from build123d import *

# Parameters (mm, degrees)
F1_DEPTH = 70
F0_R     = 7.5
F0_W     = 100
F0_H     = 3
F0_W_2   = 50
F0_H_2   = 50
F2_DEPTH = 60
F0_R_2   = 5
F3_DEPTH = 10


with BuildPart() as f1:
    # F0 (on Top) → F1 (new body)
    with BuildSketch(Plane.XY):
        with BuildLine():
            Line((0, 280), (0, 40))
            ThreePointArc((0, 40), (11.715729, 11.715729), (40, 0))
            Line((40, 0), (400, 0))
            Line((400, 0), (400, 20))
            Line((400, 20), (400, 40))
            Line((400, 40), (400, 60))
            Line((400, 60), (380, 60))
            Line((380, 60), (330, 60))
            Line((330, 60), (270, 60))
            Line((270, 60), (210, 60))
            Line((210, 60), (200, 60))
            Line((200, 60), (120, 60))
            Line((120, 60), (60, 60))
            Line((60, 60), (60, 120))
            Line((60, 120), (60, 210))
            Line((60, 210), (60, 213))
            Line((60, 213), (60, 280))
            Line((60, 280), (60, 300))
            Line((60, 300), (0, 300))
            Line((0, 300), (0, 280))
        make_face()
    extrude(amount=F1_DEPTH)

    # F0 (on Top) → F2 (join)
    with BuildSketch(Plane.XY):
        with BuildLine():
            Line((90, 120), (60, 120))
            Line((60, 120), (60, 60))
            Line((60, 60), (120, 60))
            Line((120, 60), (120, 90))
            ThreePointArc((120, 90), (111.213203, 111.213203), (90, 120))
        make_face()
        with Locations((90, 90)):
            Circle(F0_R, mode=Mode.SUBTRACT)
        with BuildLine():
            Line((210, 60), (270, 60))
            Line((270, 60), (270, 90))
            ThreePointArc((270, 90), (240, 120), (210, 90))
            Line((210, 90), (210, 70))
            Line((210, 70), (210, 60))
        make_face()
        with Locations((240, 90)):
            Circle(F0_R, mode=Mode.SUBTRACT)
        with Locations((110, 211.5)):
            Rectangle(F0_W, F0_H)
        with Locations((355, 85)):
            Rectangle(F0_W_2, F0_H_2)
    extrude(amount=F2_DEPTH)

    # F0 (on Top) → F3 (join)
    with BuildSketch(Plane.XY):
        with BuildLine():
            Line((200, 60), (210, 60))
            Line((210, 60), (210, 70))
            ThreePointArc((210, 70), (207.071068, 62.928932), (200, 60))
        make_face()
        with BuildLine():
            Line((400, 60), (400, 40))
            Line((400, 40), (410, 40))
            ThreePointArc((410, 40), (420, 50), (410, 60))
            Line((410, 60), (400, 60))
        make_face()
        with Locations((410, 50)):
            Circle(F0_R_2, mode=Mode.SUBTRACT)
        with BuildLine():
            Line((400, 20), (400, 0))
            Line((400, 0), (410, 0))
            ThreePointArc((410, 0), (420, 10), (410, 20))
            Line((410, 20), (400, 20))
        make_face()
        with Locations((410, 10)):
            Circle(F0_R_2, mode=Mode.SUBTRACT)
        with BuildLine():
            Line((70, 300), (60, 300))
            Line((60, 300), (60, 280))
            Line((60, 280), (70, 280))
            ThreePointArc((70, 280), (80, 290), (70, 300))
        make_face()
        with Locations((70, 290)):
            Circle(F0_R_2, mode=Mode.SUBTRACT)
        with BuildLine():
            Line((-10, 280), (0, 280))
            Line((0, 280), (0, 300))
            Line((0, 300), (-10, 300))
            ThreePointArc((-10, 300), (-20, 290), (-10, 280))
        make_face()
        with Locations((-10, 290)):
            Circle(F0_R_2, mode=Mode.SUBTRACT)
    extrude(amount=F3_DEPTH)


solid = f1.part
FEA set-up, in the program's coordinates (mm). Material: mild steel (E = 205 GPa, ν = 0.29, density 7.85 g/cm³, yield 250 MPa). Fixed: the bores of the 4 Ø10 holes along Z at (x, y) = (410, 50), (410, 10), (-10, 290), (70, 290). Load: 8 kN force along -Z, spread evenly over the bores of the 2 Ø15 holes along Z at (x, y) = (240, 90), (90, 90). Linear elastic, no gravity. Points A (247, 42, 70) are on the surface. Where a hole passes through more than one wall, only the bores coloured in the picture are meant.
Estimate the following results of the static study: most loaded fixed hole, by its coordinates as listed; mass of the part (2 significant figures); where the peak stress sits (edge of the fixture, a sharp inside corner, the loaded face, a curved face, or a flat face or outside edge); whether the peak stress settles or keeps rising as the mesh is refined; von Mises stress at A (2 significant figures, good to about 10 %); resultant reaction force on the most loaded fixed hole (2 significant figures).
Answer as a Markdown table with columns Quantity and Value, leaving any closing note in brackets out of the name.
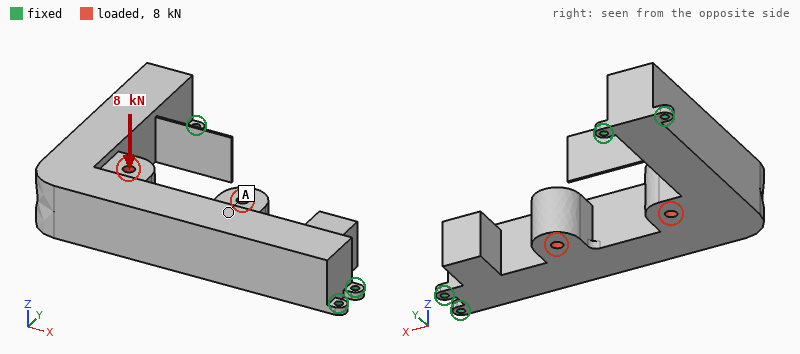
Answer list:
| Quantity | Value |
|---|---|
| most loaded fixed hole, by its coordinates as listed | (410, 10) |
| mass of the part | 25 kg |
| where the peak stress sits | edge of the fixture |
| whether the peak stress settles or keeps rising as the mesh is refined | keeps rising |
| von Mises stress at A | 14 MPa |
| resultant reaction force on the most loaded fixed hole | 13 kN |
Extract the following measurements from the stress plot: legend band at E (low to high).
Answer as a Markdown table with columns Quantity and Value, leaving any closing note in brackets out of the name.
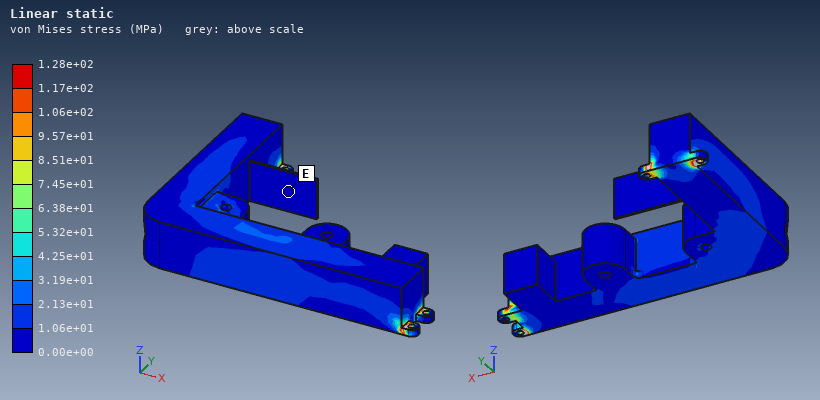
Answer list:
| Quantity | Value |
|---|---|
| legend band at E | 0.00e+00 to 1.06e+01 MPa |
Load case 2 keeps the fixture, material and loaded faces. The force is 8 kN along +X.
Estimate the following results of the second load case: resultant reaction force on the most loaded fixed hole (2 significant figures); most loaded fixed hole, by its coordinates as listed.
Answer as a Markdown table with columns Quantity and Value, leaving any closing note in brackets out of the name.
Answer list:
| Quantity | Value |
|---|---|
| resultant reaction force on the most loaded fixed hole | 4.3 kN |
| most loaded fixed hole, by its coordinates as listed | (410, 50) |
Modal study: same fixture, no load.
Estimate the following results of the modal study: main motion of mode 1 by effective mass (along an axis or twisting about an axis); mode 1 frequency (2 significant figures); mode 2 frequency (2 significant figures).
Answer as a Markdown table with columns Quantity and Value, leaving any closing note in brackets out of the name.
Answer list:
| Quantity | Value |
|---|---|
| main motion of mode 1 by effective mass | along Z |
| mode 1 frequency | 180 Hz |
| mode 2 frequency | 250 Hz |
